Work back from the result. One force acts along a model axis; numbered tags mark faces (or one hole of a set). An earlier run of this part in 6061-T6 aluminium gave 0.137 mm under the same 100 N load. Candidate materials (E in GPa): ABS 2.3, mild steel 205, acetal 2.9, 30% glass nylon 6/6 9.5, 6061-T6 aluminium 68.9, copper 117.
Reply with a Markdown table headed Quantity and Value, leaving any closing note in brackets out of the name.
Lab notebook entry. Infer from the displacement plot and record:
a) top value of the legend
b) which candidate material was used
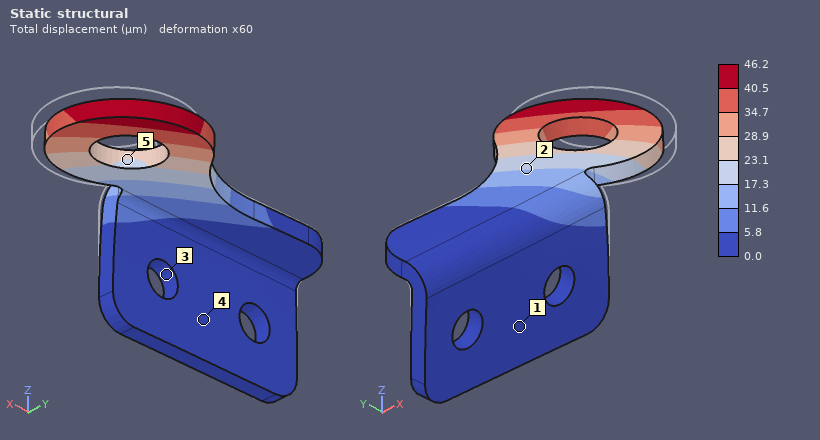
| Quantity | Value |
|---|---|
| top value of the legend | 46.2 µm |
| which candidate material was used | mild steel |
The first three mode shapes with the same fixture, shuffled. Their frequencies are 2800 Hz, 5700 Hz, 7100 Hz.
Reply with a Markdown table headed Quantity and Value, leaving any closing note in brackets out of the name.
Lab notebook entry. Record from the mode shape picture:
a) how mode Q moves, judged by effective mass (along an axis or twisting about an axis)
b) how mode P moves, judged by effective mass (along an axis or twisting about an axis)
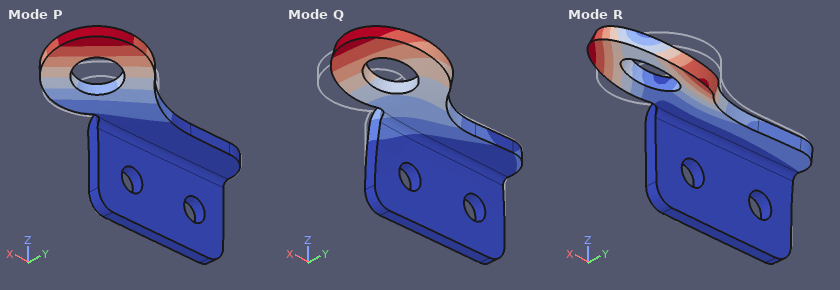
| Quantity | Value |
|---|---|
| how mode Q moves, judged by effective mass | along Y |
| how mode P moves, judged by effective mass | along Z |
